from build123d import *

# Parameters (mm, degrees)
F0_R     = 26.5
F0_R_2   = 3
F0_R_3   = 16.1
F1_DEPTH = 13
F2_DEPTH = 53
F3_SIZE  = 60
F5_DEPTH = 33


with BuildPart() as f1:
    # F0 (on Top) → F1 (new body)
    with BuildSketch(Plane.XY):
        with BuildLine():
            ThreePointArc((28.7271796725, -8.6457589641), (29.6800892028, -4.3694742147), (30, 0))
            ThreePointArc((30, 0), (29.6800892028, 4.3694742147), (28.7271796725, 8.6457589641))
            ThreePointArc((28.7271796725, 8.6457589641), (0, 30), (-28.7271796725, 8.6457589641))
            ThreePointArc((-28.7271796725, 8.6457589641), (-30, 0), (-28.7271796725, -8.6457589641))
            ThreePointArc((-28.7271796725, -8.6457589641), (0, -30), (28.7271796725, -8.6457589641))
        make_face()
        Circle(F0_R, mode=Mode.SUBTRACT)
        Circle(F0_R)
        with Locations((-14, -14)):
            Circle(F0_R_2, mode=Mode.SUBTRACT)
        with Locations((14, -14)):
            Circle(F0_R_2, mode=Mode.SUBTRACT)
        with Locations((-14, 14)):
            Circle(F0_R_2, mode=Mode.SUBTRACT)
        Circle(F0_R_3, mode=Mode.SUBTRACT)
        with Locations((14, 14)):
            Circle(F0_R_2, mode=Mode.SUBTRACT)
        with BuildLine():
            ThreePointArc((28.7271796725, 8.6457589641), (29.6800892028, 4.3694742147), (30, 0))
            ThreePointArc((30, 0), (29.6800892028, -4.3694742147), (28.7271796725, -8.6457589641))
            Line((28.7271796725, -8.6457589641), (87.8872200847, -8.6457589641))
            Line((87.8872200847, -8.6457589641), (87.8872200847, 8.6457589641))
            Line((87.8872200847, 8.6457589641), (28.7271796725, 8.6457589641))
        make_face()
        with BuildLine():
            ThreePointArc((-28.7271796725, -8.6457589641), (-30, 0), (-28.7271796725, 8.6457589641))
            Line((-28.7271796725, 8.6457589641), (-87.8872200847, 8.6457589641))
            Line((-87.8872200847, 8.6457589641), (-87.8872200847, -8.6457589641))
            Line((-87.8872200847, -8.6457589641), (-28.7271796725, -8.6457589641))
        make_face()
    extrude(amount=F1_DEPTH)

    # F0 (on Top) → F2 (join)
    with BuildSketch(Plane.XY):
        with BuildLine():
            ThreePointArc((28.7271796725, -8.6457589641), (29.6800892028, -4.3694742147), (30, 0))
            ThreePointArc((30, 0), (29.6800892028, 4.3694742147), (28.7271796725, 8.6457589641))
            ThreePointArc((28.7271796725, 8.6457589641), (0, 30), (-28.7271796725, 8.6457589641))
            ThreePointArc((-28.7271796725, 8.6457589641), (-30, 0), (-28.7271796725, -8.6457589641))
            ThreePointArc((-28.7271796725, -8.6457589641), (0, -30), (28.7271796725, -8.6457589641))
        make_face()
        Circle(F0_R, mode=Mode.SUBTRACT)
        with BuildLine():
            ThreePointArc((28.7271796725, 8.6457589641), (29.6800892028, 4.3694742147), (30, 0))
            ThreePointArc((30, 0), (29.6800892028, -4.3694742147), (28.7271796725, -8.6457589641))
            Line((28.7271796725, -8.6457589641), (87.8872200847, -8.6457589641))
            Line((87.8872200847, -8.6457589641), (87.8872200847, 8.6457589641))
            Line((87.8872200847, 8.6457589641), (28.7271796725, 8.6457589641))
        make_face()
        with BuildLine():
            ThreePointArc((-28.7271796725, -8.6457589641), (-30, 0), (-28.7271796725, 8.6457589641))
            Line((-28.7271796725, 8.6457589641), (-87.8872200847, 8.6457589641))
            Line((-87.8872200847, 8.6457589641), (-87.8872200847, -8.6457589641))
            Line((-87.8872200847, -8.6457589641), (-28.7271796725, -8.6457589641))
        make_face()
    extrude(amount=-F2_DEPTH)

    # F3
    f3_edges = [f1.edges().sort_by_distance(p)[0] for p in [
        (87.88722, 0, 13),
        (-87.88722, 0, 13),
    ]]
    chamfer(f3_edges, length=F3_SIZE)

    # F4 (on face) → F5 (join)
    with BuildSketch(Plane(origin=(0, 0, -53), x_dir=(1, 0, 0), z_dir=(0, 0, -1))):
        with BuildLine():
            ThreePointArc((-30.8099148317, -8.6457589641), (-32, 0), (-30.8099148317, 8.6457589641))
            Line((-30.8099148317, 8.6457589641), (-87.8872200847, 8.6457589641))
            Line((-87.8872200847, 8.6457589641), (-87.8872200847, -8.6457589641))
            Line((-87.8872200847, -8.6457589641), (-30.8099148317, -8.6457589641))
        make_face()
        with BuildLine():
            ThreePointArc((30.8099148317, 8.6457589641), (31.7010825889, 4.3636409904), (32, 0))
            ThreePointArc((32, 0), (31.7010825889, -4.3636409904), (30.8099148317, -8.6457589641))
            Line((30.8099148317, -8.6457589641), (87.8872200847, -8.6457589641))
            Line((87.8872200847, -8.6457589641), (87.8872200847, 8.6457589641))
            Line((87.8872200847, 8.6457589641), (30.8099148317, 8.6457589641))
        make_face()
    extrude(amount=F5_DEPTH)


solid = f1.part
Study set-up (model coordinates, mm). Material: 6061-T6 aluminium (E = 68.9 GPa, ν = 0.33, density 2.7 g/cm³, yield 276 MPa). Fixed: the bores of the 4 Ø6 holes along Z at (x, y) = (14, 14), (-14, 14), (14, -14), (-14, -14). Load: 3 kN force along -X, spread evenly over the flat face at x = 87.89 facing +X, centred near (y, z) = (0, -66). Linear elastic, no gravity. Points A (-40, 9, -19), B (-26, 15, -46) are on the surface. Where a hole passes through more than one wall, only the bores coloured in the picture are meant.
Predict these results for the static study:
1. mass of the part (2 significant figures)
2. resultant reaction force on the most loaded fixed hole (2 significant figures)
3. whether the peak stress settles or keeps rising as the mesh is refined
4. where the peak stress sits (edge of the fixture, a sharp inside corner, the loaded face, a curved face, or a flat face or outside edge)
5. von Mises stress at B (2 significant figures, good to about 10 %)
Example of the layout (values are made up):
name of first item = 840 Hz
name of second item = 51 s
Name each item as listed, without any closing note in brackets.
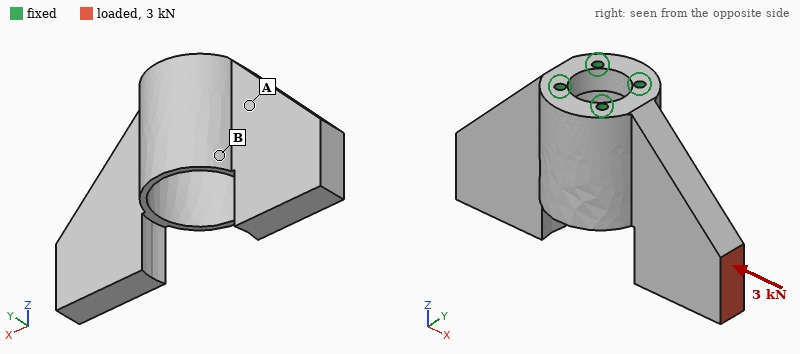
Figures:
mass of the part = 520 g
resultant reaction force on the most loaded fixed hole = 2.5 kN
whether the peak stress settles or keeps rising as the mesh is refined = keeps rising
where the peak stress sits = edge of the fixture
von Mises stress at B = 36 MPa
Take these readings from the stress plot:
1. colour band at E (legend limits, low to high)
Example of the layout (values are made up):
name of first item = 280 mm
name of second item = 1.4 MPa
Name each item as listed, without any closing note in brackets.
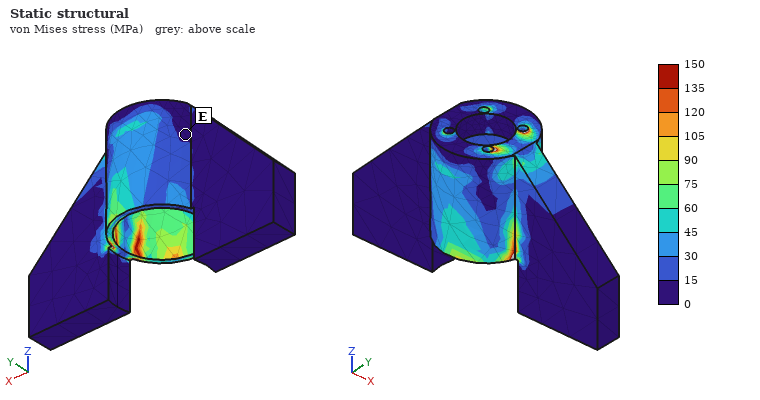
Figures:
colour band at E = 0 to 15 MPa
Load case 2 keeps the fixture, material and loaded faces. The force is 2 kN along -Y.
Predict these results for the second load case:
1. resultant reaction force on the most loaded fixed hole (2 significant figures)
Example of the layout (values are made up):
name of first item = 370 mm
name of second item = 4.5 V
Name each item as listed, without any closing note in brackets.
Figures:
resultant reaction force on the most loaded fixed hole = 4.4 kN
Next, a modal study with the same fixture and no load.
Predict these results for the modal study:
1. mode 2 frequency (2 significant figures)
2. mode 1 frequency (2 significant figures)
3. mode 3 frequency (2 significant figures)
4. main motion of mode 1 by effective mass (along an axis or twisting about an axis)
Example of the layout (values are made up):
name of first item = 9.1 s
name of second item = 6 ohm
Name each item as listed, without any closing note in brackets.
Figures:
mode 2 frequency = 1400 Hz
mode 1 frequency = 1100 Hz
mode 3 frequency = 1400 Hz
main motion of mode 1 by effective mass = along Z
